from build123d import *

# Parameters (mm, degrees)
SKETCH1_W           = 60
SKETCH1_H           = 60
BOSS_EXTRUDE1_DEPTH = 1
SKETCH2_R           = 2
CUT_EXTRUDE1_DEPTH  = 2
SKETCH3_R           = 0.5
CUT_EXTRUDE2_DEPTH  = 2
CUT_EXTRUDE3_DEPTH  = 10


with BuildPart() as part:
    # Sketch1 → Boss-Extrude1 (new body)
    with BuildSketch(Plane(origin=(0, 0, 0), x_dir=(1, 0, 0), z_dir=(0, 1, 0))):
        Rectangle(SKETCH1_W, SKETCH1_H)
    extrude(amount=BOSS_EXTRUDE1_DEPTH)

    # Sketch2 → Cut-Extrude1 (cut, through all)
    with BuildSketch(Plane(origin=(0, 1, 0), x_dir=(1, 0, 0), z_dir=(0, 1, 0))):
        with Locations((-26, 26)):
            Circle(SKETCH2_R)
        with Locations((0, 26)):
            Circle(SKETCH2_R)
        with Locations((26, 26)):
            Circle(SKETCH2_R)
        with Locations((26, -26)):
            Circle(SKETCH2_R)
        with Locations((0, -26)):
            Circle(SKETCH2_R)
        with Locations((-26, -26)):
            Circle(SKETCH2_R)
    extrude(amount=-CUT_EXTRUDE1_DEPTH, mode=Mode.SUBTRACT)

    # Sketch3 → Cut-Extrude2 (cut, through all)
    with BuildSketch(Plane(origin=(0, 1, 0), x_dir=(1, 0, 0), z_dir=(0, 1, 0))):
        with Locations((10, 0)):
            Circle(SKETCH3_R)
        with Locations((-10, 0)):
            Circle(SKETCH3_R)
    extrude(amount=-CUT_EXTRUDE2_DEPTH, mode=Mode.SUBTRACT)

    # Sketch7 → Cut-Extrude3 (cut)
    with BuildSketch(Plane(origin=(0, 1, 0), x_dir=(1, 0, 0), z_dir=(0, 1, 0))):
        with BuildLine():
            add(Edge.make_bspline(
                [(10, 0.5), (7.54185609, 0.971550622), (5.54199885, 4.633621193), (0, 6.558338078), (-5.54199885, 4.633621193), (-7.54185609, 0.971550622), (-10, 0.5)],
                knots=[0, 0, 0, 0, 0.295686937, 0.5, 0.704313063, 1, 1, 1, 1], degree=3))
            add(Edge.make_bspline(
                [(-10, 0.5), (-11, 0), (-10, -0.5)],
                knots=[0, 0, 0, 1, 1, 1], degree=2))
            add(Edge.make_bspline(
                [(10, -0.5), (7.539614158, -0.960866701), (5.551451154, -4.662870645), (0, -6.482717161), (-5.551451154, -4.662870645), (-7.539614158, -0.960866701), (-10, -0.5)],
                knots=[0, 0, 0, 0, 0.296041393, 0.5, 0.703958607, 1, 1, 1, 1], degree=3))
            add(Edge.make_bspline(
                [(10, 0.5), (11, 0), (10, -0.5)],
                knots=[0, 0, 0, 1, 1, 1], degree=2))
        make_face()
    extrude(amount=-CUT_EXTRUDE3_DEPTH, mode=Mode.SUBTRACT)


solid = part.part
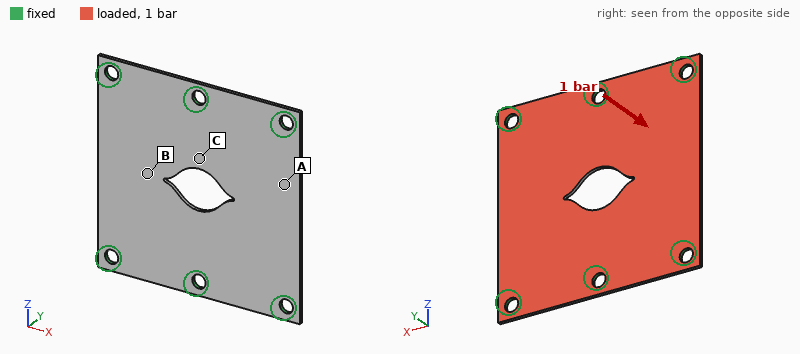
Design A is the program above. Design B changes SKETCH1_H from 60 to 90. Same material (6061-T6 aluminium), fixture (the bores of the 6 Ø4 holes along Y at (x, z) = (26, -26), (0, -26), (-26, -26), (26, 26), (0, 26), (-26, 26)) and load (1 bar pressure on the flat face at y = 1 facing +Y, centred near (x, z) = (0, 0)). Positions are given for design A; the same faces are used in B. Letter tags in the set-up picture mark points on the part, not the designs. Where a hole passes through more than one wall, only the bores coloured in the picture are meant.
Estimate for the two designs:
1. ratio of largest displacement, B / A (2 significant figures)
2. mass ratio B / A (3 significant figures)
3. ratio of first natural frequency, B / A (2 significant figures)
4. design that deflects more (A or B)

0.89
1.53
1.00
A
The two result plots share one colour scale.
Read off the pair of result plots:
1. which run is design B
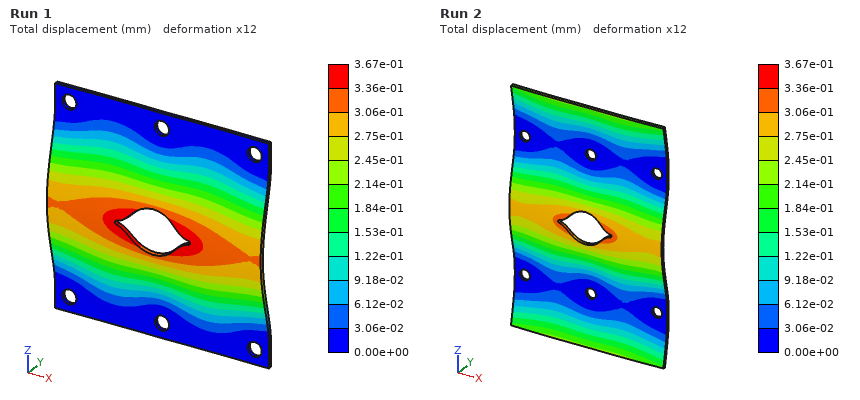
Run 2
